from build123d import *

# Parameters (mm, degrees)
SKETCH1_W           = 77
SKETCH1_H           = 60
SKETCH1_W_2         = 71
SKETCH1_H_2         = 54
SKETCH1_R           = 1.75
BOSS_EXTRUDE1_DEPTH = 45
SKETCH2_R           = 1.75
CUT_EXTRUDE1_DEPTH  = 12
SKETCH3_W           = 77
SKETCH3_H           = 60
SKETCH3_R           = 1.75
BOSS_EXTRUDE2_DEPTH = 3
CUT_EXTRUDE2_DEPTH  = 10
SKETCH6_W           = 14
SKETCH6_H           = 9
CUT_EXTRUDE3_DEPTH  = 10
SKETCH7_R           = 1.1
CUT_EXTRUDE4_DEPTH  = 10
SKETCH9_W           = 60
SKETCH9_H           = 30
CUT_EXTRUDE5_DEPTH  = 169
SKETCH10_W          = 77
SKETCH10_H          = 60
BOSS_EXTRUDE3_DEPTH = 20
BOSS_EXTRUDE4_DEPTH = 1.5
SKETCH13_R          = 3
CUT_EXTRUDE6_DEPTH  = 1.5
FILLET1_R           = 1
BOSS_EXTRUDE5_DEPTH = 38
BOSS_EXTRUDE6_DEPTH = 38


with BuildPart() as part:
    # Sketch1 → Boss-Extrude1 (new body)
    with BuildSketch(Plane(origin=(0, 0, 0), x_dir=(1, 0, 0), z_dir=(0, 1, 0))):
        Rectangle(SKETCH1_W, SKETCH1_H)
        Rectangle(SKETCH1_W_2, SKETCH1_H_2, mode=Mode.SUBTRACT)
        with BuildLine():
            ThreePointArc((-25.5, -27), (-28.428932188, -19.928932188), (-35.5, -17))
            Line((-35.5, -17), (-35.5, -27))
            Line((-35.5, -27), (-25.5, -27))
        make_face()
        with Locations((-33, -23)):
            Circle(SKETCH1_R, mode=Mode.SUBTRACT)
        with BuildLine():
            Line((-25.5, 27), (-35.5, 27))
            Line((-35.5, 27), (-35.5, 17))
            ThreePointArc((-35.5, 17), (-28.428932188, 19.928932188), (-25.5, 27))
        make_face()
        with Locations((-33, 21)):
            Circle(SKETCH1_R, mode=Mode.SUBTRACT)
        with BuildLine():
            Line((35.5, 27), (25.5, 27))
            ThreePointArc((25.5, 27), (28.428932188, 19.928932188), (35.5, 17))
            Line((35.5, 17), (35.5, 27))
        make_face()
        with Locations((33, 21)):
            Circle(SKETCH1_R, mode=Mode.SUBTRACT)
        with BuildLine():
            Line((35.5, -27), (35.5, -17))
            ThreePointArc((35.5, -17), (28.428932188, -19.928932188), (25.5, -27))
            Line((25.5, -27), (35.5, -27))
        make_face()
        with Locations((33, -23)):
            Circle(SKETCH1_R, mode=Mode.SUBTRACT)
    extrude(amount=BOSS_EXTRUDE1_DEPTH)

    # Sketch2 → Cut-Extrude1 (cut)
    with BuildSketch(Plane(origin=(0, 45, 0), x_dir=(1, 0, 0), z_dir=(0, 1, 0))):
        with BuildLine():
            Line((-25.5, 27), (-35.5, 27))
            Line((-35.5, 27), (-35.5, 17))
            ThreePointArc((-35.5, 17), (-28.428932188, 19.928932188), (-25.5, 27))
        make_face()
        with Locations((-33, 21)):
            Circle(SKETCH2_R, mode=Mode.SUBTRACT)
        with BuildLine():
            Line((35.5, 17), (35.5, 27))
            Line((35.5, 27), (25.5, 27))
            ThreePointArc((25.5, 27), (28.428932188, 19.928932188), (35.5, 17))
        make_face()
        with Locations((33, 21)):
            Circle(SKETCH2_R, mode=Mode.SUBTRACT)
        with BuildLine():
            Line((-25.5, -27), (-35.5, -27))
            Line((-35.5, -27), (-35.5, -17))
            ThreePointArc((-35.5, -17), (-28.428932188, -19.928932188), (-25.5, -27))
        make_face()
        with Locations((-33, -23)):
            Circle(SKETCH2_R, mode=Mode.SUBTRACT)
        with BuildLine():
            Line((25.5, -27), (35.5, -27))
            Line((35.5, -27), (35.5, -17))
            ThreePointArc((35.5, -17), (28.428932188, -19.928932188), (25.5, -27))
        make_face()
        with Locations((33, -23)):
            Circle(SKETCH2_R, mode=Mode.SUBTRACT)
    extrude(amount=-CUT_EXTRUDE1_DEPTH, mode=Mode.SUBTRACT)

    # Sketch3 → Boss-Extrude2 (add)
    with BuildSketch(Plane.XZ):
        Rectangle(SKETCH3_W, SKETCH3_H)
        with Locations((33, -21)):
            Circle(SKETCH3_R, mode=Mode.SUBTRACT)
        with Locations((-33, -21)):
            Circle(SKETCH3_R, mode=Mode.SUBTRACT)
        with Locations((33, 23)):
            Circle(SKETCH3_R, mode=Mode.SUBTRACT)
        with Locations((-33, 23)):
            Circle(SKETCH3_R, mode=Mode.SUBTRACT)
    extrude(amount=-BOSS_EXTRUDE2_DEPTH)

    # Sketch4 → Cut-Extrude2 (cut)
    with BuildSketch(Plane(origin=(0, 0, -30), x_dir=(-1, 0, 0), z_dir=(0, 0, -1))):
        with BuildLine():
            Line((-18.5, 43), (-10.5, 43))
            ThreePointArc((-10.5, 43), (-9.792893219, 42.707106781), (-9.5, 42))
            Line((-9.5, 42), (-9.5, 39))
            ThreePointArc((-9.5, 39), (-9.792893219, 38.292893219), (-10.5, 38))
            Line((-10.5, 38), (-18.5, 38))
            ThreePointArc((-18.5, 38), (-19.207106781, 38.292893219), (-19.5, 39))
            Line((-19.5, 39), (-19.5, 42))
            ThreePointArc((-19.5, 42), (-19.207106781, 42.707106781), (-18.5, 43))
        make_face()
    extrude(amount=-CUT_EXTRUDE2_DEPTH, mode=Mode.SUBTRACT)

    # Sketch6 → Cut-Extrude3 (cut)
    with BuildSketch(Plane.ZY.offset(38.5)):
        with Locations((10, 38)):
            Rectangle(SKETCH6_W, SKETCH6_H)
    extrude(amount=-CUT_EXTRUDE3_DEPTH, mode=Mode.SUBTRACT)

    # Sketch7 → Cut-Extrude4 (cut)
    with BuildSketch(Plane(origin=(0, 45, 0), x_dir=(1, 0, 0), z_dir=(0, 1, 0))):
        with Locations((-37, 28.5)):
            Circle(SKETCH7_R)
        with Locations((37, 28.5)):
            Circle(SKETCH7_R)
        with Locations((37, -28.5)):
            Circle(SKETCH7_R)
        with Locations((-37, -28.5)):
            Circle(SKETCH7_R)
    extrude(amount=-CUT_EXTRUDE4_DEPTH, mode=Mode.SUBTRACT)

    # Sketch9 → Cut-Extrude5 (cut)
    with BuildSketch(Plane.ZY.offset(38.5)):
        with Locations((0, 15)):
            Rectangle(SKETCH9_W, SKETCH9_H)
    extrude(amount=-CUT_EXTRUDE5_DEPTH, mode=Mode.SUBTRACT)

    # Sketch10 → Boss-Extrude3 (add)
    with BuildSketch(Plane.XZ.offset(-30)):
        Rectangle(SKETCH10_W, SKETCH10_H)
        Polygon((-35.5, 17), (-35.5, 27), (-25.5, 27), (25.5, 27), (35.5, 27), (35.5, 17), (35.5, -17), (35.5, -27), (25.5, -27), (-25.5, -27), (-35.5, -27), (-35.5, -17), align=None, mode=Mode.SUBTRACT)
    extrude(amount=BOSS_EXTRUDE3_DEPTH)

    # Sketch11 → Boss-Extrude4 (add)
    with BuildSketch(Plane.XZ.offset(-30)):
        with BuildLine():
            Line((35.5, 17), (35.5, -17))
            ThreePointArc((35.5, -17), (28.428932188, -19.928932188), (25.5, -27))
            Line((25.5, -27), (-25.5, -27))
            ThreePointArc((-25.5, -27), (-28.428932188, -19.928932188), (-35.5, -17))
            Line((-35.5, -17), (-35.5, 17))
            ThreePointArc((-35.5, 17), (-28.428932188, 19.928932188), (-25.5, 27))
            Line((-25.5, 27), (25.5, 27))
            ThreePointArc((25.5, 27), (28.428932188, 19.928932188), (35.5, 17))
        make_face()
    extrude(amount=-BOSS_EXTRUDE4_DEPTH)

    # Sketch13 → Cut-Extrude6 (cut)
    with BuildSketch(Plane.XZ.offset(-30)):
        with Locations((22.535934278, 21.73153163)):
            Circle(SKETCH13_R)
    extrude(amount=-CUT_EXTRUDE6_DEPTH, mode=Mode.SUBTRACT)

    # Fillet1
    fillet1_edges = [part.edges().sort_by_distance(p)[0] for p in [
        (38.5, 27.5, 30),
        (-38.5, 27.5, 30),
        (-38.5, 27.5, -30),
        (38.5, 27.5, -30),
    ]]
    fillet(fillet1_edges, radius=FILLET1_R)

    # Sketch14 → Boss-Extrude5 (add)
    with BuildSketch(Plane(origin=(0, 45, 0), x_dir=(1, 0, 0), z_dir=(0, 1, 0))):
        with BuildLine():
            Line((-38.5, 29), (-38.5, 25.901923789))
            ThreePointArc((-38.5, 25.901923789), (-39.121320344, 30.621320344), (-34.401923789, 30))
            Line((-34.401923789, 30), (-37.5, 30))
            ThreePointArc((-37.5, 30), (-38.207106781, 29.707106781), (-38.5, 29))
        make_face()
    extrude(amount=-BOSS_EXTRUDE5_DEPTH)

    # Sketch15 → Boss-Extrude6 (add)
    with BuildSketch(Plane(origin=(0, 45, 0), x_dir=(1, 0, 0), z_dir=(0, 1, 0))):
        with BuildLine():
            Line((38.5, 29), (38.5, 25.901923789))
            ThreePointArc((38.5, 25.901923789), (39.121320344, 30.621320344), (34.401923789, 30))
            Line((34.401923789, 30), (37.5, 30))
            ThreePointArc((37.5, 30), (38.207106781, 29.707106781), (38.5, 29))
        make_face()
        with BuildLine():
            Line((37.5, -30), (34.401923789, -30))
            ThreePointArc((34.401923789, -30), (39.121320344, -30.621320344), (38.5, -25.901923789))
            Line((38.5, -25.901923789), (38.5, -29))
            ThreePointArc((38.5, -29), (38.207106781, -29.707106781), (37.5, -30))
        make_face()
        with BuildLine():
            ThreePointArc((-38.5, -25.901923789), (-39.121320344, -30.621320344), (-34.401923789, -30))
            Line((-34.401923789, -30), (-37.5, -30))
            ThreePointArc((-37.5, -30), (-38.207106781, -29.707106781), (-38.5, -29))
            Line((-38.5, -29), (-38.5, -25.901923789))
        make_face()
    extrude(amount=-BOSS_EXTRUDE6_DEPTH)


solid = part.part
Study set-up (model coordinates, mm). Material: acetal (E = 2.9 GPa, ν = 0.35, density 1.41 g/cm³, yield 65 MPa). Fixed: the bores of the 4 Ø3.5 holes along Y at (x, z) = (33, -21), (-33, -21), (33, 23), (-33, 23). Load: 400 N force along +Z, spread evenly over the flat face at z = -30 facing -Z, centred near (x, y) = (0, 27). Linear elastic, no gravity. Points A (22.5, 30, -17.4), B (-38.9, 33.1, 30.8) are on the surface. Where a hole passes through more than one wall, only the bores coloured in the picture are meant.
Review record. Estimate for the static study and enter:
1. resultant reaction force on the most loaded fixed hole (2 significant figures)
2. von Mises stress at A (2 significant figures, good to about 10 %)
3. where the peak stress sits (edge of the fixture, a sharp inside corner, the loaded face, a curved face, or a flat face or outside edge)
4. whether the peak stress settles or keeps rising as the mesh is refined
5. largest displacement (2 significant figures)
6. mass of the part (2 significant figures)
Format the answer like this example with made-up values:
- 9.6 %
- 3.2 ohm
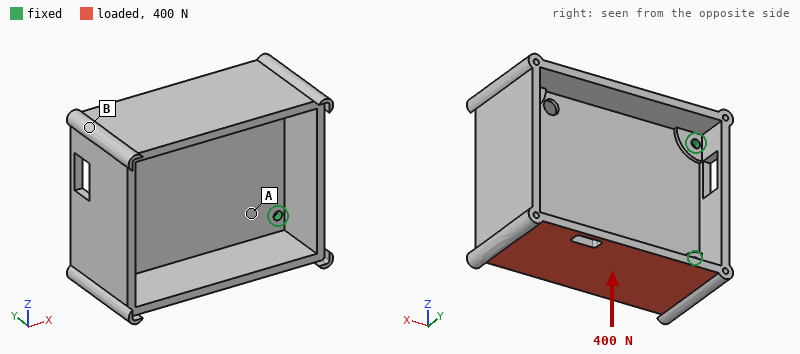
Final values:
- 130 N
- 3.4 MPa
- edge of the fixture
- keeps rising
- 0.74 mm
- 49 g
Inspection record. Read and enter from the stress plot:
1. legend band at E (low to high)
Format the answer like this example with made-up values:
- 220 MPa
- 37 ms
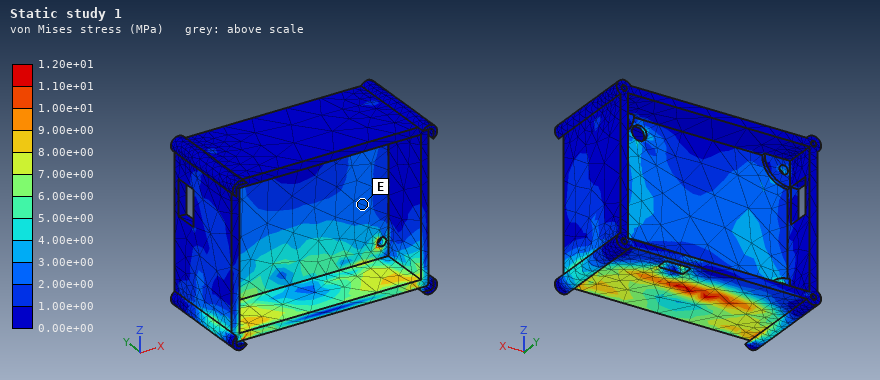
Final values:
- 2.00e+00 to 3.00e+00 MPa
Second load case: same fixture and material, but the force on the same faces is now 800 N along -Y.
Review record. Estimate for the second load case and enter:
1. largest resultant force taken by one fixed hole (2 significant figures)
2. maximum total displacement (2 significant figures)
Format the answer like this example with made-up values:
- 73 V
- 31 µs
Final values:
- 480 N
- 0.63 mm
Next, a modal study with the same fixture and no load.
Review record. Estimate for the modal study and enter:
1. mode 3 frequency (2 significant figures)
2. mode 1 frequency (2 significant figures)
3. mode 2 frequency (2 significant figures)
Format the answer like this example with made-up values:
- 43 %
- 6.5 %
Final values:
- 1300 Hz
- 940 Hz
- 1300 Hz
